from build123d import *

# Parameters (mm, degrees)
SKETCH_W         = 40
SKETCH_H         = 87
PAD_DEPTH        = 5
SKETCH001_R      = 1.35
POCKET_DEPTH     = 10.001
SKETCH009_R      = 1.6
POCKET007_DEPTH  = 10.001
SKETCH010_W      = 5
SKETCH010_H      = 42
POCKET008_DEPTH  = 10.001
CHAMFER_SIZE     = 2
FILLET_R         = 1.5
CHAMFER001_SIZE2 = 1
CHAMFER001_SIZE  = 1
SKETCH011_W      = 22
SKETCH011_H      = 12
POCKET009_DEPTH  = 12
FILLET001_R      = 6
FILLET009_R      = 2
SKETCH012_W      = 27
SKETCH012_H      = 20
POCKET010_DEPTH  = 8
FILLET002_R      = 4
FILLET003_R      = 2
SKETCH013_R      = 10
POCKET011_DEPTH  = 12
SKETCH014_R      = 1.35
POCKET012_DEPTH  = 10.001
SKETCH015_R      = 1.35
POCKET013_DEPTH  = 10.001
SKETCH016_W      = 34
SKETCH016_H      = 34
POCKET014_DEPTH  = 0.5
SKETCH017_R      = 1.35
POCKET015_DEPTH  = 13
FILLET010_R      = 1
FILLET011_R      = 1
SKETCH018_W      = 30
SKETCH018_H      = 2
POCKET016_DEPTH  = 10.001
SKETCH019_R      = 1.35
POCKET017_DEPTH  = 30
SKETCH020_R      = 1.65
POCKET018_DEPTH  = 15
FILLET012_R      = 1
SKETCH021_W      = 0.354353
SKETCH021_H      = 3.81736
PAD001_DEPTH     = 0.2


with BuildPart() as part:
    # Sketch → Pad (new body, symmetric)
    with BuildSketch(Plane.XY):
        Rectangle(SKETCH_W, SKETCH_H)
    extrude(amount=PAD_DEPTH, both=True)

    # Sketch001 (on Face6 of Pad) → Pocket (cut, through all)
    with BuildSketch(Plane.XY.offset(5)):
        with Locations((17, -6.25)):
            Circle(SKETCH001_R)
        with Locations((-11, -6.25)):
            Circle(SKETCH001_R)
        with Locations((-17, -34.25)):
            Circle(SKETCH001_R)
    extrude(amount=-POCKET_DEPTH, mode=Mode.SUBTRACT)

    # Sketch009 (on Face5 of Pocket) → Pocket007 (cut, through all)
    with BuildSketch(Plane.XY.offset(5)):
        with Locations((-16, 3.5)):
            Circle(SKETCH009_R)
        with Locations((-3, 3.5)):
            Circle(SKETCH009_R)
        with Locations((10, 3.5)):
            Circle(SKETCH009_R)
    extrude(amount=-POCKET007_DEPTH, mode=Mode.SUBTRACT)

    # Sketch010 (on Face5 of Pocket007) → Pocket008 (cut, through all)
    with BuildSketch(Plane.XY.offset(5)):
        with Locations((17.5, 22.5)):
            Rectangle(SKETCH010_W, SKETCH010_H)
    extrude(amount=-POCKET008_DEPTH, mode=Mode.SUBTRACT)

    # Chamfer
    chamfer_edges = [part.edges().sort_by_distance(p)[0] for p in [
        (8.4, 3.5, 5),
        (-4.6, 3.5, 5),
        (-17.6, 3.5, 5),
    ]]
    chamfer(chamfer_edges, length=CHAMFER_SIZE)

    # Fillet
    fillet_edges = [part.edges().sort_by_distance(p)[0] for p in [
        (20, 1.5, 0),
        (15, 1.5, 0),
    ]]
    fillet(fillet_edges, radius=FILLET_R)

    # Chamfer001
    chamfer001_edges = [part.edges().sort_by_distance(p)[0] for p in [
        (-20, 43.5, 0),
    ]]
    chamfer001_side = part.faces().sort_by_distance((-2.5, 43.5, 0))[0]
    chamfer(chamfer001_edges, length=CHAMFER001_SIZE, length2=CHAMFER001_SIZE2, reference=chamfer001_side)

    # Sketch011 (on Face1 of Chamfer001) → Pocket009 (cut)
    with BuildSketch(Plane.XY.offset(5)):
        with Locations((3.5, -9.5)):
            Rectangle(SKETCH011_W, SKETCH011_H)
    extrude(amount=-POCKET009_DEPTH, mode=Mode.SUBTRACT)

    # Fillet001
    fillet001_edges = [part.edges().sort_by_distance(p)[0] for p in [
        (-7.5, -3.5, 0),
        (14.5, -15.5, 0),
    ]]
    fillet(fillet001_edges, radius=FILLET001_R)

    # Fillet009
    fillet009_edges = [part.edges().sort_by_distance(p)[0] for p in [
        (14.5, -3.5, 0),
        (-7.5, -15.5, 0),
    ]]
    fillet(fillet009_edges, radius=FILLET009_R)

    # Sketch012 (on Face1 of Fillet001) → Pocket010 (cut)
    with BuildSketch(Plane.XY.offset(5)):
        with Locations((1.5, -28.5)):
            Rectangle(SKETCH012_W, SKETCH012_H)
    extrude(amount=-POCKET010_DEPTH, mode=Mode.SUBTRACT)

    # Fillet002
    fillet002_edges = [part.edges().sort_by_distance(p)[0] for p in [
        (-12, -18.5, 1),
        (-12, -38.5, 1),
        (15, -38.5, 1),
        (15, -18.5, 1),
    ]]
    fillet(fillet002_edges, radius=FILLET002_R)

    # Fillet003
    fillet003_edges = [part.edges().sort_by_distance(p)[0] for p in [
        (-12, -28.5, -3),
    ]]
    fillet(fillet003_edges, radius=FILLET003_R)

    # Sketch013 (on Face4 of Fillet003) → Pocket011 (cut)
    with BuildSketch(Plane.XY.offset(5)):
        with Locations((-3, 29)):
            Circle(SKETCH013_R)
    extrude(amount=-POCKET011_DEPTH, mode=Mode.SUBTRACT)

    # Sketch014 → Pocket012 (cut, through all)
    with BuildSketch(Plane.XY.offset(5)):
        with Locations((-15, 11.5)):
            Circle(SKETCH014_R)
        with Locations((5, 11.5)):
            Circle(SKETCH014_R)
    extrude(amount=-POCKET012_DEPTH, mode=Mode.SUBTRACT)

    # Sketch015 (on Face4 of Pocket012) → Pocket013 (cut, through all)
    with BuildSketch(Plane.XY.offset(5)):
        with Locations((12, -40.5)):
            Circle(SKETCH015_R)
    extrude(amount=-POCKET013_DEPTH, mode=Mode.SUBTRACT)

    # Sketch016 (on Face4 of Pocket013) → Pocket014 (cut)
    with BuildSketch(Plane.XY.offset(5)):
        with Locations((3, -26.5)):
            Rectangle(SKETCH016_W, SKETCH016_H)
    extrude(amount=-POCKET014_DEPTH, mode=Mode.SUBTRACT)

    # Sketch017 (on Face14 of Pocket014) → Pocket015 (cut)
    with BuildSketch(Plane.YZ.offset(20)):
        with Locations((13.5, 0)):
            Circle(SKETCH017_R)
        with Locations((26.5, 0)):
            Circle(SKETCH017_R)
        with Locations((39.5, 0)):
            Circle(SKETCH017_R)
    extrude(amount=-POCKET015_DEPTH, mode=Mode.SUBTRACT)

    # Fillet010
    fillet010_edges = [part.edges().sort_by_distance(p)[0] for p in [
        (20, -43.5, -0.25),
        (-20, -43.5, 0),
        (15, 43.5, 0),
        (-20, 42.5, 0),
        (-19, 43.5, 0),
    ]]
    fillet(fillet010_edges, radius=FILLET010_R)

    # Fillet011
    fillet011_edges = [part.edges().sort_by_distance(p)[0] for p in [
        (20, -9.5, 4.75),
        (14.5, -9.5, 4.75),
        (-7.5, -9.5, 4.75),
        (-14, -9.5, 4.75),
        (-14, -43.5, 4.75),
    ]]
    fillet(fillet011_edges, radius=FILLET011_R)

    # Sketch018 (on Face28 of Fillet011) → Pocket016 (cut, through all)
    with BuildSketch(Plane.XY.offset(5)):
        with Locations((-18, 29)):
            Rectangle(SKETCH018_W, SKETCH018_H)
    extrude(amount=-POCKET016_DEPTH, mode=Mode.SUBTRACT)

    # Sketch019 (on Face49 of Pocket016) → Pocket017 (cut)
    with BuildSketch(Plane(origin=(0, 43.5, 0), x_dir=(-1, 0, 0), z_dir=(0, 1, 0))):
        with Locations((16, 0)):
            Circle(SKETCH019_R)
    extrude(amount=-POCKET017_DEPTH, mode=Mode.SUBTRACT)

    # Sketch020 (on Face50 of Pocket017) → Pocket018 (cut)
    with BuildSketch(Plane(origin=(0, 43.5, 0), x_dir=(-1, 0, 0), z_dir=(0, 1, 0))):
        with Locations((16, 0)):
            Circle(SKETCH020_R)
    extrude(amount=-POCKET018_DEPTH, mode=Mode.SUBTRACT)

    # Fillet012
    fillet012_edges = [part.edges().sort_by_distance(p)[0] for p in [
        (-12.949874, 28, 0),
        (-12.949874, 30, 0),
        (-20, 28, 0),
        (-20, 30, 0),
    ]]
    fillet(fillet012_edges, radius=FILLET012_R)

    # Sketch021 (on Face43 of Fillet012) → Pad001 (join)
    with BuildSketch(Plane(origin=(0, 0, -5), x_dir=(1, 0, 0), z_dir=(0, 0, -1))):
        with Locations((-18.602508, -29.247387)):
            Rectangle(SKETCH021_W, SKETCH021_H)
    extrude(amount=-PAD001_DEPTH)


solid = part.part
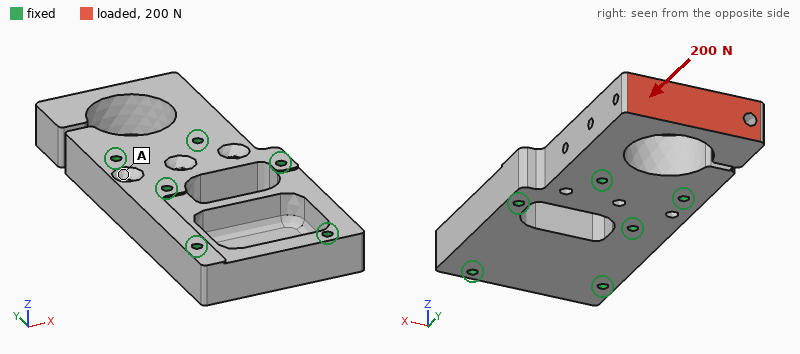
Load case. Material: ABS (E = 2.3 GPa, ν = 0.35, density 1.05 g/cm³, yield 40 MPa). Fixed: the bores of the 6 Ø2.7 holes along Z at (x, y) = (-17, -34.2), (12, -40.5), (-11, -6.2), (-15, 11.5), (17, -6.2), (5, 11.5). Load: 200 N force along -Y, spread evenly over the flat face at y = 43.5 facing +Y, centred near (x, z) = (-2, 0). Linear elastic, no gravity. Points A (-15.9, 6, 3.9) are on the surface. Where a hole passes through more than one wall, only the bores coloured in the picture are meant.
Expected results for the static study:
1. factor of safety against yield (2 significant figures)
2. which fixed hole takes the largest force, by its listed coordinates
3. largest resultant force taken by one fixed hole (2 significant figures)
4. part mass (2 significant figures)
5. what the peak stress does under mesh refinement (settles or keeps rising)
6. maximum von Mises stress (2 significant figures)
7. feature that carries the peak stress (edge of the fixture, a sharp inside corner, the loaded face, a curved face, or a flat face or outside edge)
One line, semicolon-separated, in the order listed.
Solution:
0.061; (5, 11.5); 130 N; 23 g; settles; 660 MPa; a flat face or outside edge
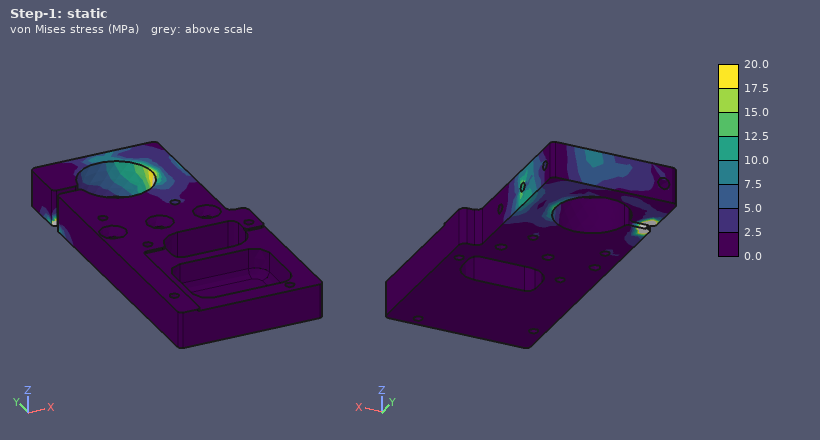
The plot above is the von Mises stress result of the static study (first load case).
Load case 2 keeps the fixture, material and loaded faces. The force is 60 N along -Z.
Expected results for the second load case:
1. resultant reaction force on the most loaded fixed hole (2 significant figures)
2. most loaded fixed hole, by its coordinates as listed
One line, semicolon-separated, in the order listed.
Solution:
83 N; (5, 11.5)
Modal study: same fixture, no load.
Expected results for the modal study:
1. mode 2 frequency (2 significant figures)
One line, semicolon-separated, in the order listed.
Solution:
1300 Hz
